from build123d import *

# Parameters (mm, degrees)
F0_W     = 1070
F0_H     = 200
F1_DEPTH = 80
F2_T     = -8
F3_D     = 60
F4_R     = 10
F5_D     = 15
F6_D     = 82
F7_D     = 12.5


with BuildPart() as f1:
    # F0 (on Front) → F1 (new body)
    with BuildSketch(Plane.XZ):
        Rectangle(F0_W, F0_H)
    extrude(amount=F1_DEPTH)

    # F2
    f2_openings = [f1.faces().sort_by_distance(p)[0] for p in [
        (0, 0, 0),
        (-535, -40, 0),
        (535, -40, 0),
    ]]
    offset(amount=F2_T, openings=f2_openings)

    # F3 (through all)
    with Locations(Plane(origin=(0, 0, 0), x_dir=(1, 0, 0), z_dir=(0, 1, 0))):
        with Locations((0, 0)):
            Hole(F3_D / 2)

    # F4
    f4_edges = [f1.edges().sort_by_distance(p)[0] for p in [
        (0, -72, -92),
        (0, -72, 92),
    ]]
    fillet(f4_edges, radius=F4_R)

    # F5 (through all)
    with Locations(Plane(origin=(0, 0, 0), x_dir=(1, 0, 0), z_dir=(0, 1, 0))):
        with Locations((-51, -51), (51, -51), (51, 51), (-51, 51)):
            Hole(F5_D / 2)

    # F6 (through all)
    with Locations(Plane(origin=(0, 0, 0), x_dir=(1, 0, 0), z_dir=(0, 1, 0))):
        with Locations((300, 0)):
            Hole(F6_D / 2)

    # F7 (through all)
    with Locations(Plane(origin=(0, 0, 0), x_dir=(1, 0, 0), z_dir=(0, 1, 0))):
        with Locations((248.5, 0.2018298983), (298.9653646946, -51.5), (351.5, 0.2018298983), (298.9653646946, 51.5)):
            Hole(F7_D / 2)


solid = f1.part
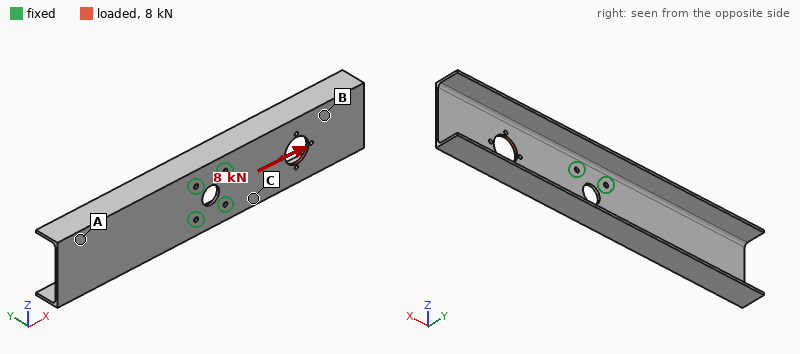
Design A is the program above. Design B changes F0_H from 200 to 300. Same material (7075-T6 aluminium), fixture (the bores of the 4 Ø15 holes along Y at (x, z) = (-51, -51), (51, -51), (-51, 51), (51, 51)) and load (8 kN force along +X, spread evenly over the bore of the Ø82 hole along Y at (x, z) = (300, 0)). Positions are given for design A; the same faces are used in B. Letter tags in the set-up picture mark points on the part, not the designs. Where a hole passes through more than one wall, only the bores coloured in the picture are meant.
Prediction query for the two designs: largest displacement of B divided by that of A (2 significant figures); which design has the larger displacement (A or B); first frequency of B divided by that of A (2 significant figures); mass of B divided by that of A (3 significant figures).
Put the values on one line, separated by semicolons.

0.55; A; 0.53; 1.29
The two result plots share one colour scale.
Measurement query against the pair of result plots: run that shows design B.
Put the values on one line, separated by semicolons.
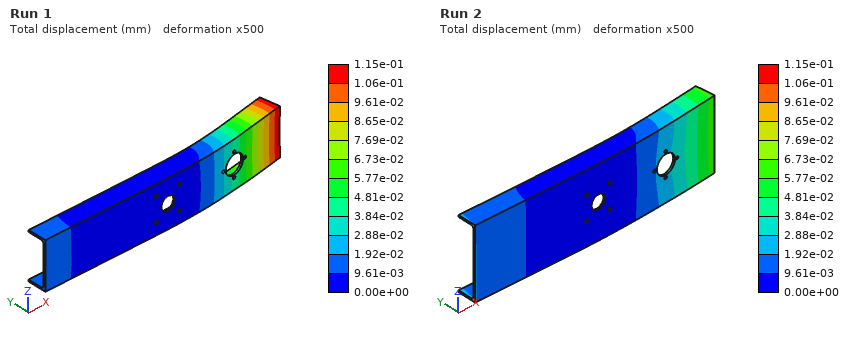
Run 2
